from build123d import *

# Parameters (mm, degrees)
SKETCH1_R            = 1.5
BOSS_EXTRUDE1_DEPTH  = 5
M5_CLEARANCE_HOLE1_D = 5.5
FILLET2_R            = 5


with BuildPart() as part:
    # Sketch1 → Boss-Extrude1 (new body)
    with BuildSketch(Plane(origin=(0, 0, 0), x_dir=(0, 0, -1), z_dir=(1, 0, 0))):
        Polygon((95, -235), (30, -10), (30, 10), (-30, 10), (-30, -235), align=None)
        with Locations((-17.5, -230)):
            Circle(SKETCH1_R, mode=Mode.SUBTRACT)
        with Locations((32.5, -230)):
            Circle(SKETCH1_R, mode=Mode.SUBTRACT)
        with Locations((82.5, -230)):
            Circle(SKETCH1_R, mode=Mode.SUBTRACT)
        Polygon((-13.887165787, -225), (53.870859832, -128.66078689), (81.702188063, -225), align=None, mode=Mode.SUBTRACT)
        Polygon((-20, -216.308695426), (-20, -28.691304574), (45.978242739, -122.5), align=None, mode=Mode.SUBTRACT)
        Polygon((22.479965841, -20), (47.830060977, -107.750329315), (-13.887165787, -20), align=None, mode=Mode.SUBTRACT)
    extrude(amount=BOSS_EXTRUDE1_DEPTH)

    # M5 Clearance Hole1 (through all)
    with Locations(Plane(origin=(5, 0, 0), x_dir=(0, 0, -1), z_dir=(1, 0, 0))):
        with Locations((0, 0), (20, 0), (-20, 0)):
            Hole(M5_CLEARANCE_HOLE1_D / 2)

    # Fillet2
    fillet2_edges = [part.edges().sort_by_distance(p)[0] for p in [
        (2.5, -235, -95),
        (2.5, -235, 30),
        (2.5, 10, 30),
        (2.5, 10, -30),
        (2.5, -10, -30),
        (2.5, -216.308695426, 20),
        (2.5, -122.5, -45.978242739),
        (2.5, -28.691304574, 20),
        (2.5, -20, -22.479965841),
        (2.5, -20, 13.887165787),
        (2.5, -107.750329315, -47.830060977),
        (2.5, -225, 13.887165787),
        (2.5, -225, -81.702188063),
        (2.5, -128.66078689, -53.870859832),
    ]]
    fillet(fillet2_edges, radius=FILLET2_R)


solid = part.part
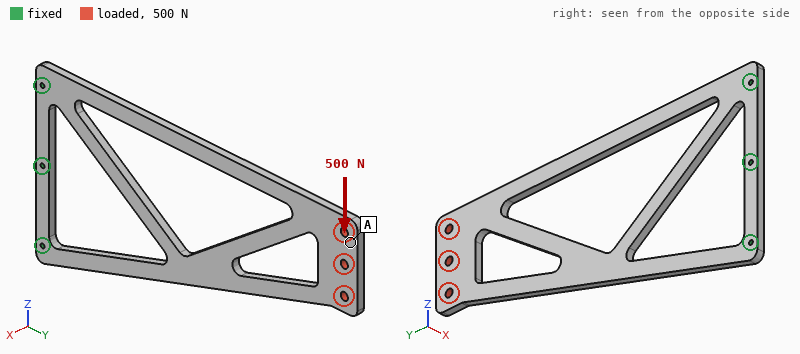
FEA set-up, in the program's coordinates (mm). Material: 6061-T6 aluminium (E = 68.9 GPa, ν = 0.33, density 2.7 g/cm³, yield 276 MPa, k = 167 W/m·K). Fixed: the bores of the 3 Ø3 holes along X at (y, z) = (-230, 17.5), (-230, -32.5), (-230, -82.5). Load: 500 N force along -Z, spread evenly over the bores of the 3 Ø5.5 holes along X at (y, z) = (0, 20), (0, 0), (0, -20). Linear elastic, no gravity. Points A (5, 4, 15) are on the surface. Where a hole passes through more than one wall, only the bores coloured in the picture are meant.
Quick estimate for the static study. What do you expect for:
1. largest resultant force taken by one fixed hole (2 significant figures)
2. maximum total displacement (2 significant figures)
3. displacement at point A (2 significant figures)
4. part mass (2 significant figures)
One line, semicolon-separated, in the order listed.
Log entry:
1.1 kN; 0.23 mm; 0.22 mm; 130 g
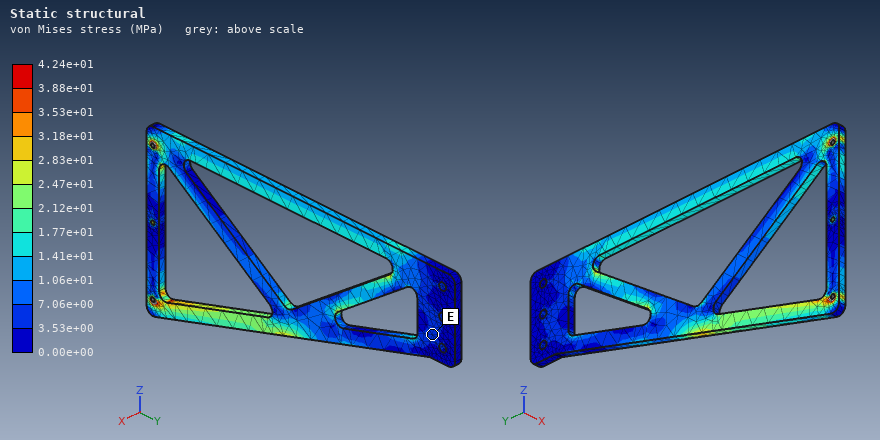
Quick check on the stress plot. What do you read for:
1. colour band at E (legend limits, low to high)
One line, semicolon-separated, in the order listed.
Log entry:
3.53e+00 to 7.06e+00 MPa
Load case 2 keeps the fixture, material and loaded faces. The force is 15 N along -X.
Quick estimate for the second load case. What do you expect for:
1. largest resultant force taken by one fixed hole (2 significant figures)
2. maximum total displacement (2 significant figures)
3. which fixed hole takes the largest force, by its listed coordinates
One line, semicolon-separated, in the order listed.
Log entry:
17 N; 3.2 mm; (-230, 17.5)
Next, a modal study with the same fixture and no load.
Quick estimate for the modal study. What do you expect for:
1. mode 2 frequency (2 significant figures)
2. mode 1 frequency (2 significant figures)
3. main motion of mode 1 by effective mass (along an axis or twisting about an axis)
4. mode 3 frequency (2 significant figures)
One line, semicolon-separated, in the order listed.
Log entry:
310 Hz; 57 Hz; along X; 410 Hz
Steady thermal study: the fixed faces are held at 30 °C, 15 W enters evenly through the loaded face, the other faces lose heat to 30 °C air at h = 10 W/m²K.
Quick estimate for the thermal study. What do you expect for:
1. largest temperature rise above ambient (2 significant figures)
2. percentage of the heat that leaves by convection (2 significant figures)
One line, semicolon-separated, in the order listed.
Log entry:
77 K; 61 %
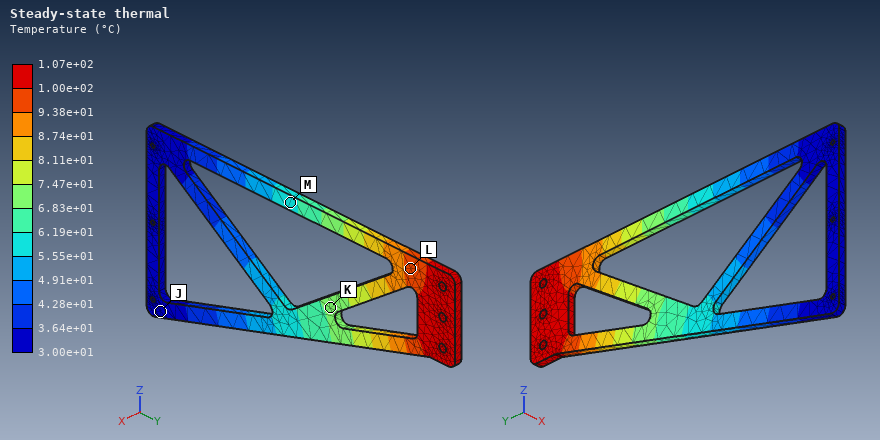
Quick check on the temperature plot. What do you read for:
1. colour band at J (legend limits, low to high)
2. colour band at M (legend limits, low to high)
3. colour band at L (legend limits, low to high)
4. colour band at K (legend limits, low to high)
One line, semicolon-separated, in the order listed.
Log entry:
3.00e+01 to 3.64e+01 °C; 5.55e+01 to 6.19e+01 °C; 9.38e+01 to 1.00e+02 °C; 6.83e+01 to 7.47e+01 °C
